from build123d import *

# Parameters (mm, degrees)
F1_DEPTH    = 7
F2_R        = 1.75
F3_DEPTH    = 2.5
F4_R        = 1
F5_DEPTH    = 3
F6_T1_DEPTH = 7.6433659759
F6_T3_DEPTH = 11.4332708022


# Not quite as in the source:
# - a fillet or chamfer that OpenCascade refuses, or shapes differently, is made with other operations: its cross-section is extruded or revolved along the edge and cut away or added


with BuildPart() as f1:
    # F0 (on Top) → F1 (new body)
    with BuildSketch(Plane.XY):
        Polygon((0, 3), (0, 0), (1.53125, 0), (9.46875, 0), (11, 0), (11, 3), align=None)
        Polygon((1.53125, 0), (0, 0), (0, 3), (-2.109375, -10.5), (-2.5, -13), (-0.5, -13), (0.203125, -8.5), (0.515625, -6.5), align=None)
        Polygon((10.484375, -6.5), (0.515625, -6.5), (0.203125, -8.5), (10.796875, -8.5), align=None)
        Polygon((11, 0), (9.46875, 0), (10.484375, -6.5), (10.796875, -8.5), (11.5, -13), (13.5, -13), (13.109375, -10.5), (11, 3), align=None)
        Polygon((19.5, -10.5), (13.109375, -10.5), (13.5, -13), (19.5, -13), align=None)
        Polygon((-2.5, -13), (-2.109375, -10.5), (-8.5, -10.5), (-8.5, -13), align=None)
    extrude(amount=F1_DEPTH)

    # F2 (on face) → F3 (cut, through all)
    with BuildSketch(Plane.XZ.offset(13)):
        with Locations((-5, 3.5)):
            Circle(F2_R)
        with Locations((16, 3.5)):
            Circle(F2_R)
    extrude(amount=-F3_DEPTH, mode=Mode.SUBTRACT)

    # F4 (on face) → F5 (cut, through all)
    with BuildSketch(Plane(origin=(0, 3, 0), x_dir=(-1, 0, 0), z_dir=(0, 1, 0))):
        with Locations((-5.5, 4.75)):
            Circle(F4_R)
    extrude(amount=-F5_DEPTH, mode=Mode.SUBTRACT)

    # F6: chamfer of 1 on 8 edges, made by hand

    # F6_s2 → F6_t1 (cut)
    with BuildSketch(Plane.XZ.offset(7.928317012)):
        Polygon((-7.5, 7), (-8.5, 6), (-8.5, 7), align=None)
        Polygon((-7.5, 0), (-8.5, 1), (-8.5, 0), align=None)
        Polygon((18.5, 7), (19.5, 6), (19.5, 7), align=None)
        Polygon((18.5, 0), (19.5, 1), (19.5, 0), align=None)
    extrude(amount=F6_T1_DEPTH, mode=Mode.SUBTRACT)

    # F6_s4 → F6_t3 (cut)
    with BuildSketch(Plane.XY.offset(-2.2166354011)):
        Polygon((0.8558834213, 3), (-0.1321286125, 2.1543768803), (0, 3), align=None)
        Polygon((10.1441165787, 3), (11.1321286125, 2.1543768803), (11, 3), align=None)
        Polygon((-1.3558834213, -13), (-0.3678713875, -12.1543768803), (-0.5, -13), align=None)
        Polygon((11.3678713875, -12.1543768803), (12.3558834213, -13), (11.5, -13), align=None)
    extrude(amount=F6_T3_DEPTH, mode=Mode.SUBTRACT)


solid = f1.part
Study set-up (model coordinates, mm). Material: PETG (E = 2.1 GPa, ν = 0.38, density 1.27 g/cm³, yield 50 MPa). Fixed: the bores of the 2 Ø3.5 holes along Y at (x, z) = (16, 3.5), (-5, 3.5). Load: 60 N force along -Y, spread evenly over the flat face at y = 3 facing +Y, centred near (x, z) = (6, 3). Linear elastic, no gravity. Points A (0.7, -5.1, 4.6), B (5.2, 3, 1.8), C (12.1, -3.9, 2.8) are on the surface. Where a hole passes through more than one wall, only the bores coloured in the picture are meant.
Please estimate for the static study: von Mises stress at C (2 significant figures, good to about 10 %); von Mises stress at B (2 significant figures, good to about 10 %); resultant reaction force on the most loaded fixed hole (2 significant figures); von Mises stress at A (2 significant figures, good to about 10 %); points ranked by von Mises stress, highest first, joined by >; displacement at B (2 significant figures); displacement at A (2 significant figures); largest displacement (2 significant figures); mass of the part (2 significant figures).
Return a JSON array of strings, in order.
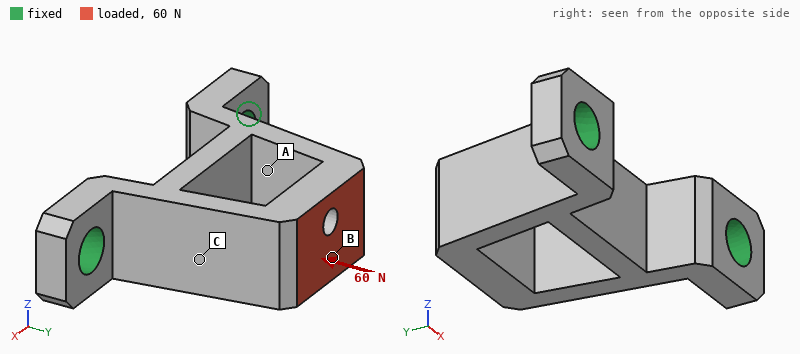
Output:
["1.2 MPa", "5.3 MPa", "32 N", "2.9 MPa", "B > A > C", "42 µm", "15 µm", "45 µm", "1.1 g"]
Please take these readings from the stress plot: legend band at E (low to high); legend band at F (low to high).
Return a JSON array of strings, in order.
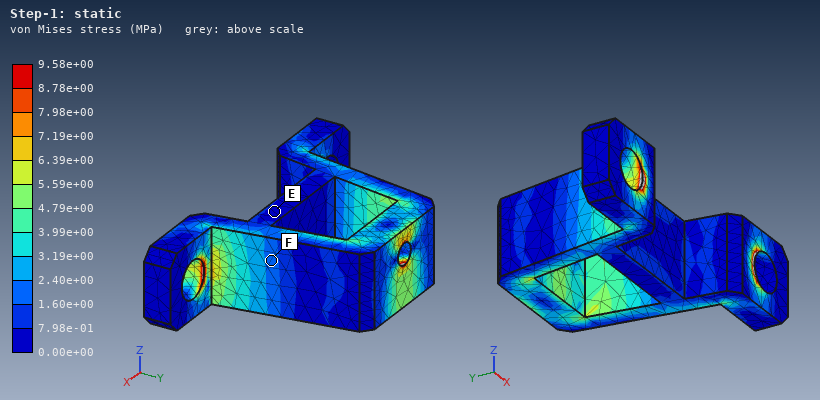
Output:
["0.00e+00 to 7.98e-01 MPa", "1.60e+00 to 2.40e+00 MPa"]
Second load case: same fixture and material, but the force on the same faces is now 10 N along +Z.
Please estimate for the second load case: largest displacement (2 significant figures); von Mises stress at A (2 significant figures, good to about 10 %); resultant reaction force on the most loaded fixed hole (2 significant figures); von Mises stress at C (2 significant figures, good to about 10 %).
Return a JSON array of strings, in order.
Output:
["0.14 mm", "1.3 MPa", "5.0 N", "0.91 MPa"]
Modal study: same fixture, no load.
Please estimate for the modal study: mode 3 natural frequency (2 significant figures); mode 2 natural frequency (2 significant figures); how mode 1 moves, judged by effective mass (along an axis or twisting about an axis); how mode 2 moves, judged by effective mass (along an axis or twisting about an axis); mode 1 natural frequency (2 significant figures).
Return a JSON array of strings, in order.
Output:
["5400 Hz", "3800 Hz", "along Z", "along X", "2400 Hz"]
